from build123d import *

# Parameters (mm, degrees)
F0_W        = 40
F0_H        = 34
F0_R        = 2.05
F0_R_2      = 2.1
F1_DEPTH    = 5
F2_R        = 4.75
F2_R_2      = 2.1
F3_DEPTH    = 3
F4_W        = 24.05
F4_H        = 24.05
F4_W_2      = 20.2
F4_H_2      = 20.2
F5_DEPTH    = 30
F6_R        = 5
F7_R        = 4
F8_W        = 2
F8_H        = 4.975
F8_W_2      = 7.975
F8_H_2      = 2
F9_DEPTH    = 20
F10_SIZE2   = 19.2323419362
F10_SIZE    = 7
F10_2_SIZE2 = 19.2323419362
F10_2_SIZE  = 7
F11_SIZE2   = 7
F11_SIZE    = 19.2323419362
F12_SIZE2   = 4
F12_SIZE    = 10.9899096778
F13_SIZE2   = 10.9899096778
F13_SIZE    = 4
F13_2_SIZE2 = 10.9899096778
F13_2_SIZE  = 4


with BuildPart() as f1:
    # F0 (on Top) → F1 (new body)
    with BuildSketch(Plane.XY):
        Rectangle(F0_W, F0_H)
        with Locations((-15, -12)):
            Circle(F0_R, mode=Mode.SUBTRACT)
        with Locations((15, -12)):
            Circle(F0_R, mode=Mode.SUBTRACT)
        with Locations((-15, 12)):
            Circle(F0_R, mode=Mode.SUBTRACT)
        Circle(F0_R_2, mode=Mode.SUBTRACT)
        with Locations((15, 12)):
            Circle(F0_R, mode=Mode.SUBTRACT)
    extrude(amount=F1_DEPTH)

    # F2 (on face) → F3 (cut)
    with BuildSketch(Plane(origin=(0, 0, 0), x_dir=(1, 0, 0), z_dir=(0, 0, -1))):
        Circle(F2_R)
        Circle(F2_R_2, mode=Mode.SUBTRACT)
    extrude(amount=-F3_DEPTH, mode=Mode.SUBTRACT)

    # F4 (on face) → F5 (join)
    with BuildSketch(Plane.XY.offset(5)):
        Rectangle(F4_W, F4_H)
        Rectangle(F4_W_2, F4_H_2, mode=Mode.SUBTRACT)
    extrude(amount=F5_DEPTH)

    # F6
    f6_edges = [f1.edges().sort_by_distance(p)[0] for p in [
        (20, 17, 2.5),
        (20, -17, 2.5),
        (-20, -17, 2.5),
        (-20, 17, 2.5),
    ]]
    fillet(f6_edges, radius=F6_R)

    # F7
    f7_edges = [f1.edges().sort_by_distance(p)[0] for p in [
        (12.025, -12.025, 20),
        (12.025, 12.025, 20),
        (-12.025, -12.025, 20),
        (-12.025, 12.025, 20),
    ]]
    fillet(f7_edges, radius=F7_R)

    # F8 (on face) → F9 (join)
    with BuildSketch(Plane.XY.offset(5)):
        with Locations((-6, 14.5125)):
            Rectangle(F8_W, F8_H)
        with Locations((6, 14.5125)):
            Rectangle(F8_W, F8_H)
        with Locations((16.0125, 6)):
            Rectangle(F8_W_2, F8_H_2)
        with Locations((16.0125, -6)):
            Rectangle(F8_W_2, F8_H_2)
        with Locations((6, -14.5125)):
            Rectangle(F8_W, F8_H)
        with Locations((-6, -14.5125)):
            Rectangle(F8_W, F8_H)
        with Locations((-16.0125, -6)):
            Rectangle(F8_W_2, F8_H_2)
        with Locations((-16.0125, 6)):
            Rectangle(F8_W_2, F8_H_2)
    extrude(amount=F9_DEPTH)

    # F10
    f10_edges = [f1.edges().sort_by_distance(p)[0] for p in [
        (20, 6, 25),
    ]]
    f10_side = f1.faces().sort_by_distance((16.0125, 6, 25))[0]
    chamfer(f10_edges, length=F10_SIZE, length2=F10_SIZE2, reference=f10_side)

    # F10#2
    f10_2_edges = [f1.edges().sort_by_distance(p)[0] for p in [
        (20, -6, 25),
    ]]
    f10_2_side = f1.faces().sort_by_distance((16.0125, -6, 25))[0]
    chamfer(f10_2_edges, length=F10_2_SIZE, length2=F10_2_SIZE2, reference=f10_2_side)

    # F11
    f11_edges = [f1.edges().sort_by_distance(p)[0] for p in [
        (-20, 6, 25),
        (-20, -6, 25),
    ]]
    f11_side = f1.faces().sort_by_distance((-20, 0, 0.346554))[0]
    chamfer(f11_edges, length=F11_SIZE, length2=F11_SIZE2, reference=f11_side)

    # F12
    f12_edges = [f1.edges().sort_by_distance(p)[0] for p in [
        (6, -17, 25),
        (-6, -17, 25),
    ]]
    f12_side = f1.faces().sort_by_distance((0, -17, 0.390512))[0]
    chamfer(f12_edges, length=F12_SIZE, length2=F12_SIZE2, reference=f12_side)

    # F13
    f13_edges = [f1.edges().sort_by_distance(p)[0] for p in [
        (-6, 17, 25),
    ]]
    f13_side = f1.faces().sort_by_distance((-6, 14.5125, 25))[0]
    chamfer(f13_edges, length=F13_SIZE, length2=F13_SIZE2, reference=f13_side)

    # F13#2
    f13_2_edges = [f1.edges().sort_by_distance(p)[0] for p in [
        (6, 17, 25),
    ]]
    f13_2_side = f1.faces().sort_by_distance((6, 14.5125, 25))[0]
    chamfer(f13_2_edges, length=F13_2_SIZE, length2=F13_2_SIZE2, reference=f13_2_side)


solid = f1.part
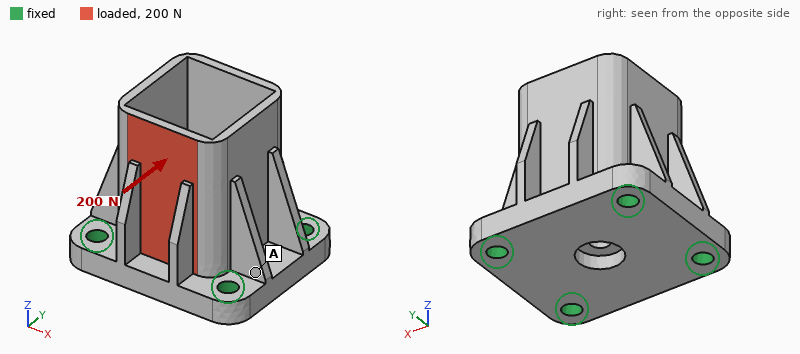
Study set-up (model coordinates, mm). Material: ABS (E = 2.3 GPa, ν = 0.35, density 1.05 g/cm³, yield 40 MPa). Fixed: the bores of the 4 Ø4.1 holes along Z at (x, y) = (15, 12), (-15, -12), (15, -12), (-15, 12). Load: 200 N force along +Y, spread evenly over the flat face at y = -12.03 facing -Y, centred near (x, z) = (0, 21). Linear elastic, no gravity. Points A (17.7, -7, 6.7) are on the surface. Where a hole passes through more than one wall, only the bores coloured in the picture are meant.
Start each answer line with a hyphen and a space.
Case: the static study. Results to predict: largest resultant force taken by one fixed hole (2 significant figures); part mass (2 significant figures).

- 95 N
- 13 g
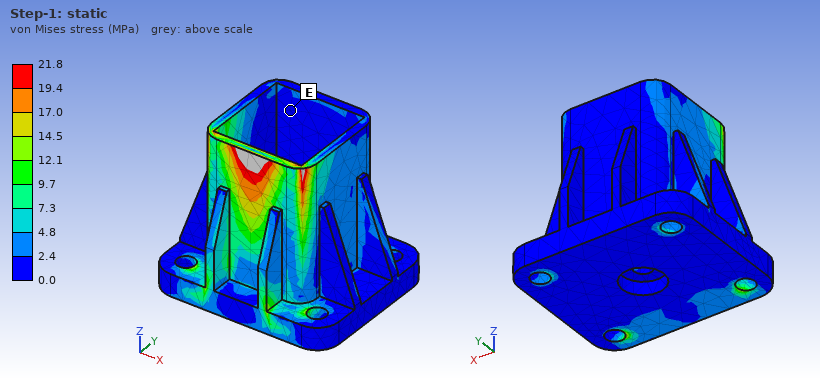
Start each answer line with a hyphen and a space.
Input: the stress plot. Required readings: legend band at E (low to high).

- 0.0 to 2.4 MPa
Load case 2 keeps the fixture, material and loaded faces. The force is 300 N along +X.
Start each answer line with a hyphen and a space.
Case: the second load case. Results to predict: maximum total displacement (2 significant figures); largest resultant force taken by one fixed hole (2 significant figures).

- 0.25 mm
- 220 N
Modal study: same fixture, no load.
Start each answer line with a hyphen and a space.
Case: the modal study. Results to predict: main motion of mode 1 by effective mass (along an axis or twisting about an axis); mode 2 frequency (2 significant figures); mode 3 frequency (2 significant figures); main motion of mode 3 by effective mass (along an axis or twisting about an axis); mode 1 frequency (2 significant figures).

- along Y
- 3300 Hz
- 3800 Hz
- along X
- 3200 Hz
